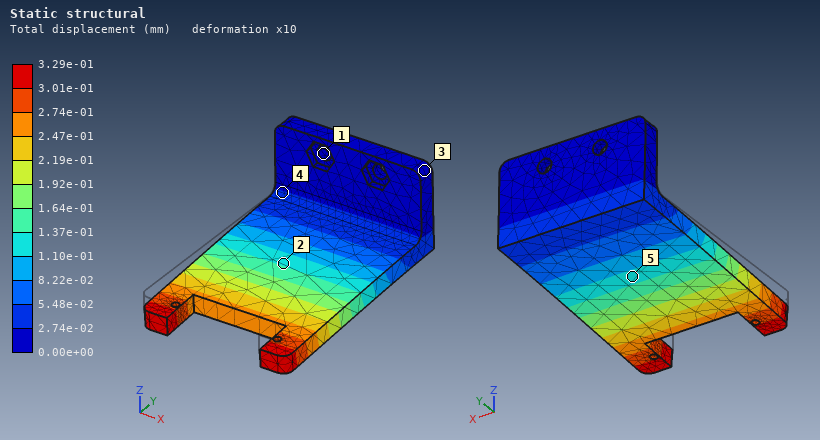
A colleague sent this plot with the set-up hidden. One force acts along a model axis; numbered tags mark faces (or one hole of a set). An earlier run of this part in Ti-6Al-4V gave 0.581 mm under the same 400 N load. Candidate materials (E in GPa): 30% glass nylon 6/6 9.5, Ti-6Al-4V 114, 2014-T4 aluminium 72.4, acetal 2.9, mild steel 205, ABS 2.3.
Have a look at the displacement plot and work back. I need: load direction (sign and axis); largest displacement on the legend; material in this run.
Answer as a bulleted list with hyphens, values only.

- -Z
- 3.29e-01 mm
- mild steel
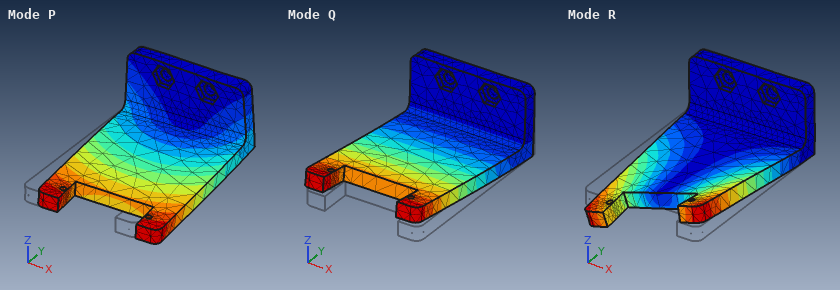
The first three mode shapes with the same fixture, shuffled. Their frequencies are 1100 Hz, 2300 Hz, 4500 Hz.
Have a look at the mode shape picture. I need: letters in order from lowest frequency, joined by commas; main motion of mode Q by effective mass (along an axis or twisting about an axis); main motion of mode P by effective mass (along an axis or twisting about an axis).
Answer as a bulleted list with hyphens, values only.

- Q, P, R
- along Z
- along X
